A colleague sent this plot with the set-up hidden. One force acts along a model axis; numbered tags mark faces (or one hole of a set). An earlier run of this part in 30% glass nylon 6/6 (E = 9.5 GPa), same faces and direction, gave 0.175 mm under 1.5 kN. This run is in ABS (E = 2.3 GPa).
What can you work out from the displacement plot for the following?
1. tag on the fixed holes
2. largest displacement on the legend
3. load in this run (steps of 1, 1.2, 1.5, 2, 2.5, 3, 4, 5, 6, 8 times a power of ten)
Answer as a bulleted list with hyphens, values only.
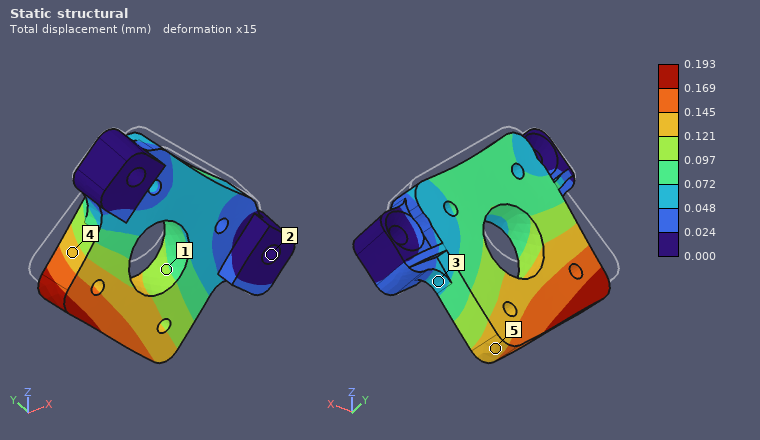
- 2
- 0.193 mm
- 400 N
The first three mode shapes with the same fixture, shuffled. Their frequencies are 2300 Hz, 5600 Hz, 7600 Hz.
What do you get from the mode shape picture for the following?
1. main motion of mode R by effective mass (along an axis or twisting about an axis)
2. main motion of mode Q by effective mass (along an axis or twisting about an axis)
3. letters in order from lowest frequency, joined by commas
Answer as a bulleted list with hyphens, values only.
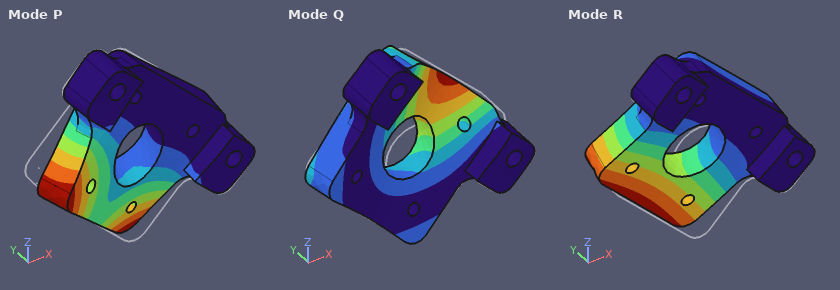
- along Y
- along Y
- R, P, Q
